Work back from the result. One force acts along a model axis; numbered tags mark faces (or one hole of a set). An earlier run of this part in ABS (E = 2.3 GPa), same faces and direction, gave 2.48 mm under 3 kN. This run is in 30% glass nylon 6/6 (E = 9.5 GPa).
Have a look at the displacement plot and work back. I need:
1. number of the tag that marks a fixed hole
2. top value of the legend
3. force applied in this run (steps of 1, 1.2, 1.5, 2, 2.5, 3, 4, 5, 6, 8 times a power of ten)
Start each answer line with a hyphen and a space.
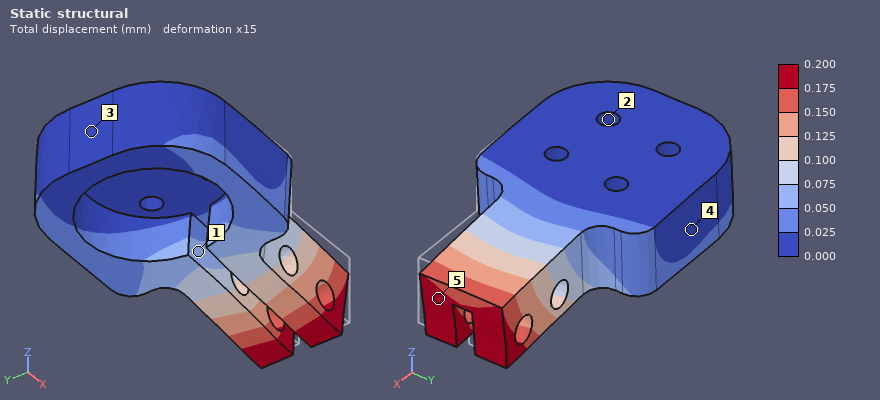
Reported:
- 2
- 0.200 mm
- 1 kN
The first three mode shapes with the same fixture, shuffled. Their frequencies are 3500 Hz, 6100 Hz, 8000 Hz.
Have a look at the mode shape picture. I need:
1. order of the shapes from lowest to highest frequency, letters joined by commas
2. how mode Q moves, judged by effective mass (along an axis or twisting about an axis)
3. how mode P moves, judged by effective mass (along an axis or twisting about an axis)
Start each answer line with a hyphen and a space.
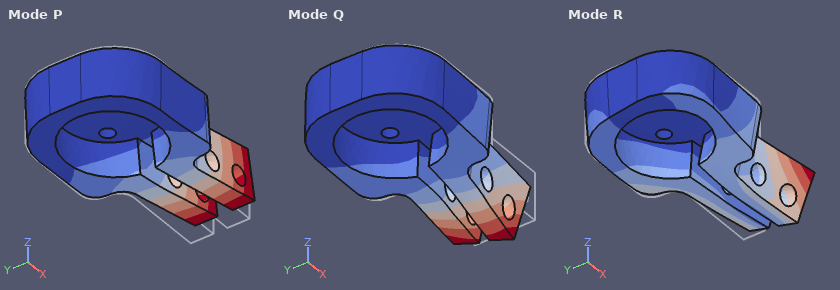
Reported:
- P, Q, R
- along Y
- along Z
